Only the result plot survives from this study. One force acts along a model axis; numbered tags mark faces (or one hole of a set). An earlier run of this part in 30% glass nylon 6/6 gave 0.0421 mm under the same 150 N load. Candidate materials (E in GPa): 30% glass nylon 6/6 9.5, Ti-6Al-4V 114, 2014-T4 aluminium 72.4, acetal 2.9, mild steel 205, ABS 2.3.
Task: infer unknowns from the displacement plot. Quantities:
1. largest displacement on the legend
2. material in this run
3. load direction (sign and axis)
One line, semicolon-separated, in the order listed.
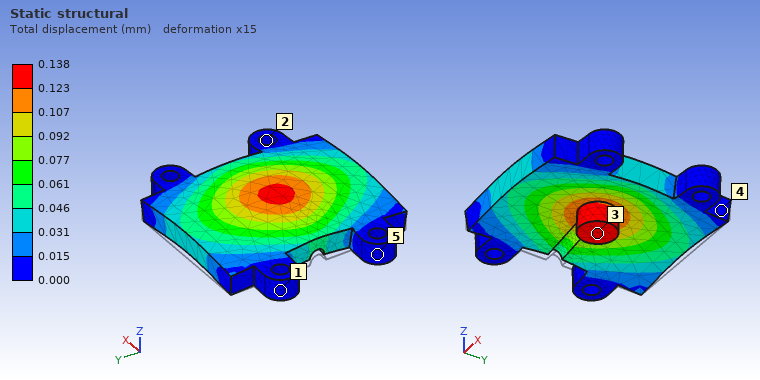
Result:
0.138 mm; acetal; +Z
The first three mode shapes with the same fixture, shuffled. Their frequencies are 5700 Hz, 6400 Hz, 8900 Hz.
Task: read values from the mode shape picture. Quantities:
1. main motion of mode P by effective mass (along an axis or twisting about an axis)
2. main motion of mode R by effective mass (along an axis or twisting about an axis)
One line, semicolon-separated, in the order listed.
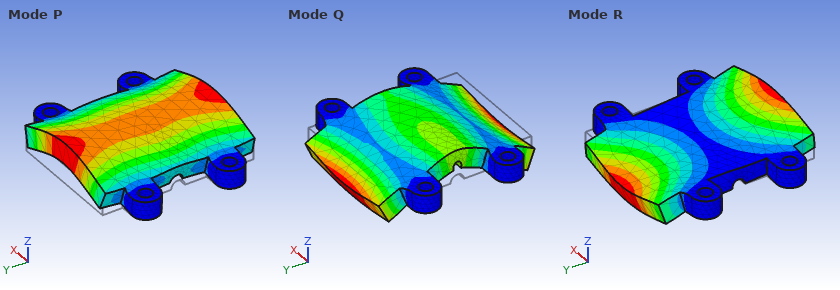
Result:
along Z; twisting about X
